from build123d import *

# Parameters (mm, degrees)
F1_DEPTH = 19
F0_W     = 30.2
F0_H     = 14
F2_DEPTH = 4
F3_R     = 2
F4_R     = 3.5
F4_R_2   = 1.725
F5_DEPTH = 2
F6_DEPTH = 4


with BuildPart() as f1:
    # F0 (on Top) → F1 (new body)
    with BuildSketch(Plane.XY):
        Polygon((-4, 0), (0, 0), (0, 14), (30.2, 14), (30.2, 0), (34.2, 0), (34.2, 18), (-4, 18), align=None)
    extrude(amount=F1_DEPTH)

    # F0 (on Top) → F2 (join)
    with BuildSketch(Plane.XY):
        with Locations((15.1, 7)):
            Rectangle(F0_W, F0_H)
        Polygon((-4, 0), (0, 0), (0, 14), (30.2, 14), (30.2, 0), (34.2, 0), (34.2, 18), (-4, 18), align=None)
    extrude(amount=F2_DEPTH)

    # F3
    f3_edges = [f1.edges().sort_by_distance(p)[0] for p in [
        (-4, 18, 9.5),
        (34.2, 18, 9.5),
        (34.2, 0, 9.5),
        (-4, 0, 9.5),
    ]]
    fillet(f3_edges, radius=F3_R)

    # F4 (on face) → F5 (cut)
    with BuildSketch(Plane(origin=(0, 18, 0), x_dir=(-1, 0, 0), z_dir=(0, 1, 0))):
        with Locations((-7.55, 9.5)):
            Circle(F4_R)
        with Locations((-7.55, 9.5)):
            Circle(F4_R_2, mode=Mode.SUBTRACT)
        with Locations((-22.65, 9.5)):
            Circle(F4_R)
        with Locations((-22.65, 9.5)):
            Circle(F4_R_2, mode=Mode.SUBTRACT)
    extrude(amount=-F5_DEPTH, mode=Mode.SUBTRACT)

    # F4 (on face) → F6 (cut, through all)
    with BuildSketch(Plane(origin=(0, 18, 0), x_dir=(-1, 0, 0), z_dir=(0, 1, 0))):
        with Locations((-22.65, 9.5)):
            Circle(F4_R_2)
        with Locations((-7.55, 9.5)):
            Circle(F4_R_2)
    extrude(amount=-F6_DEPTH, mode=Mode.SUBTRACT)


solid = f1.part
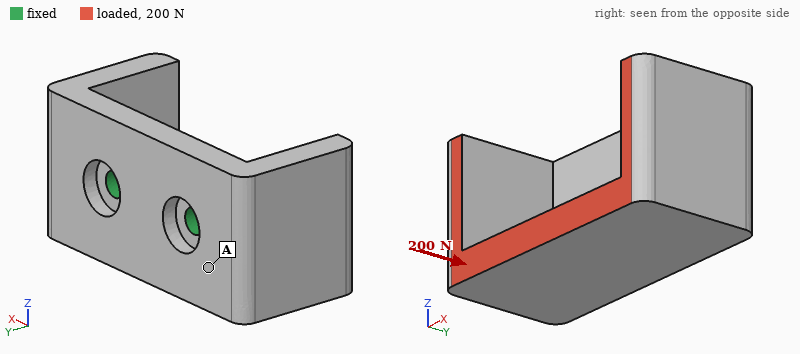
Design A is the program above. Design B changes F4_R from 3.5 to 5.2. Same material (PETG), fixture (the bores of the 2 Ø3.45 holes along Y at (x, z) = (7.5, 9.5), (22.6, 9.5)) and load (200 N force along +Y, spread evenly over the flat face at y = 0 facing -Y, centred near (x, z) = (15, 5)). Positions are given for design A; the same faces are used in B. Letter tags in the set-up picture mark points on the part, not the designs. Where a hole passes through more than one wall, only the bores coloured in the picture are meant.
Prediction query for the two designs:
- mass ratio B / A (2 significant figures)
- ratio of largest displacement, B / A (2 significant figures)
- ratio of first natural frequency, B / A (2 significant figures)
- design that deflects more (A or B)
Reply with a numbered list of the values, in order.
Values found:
1. 0.97
2. 1.1
3. 0.94
4. B
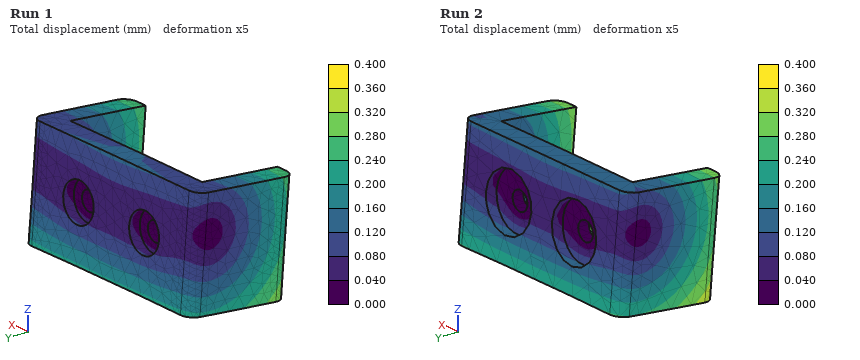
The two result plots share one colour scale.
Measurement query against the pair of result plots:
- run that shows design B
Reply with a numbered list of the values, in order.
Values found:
1. Run 2
